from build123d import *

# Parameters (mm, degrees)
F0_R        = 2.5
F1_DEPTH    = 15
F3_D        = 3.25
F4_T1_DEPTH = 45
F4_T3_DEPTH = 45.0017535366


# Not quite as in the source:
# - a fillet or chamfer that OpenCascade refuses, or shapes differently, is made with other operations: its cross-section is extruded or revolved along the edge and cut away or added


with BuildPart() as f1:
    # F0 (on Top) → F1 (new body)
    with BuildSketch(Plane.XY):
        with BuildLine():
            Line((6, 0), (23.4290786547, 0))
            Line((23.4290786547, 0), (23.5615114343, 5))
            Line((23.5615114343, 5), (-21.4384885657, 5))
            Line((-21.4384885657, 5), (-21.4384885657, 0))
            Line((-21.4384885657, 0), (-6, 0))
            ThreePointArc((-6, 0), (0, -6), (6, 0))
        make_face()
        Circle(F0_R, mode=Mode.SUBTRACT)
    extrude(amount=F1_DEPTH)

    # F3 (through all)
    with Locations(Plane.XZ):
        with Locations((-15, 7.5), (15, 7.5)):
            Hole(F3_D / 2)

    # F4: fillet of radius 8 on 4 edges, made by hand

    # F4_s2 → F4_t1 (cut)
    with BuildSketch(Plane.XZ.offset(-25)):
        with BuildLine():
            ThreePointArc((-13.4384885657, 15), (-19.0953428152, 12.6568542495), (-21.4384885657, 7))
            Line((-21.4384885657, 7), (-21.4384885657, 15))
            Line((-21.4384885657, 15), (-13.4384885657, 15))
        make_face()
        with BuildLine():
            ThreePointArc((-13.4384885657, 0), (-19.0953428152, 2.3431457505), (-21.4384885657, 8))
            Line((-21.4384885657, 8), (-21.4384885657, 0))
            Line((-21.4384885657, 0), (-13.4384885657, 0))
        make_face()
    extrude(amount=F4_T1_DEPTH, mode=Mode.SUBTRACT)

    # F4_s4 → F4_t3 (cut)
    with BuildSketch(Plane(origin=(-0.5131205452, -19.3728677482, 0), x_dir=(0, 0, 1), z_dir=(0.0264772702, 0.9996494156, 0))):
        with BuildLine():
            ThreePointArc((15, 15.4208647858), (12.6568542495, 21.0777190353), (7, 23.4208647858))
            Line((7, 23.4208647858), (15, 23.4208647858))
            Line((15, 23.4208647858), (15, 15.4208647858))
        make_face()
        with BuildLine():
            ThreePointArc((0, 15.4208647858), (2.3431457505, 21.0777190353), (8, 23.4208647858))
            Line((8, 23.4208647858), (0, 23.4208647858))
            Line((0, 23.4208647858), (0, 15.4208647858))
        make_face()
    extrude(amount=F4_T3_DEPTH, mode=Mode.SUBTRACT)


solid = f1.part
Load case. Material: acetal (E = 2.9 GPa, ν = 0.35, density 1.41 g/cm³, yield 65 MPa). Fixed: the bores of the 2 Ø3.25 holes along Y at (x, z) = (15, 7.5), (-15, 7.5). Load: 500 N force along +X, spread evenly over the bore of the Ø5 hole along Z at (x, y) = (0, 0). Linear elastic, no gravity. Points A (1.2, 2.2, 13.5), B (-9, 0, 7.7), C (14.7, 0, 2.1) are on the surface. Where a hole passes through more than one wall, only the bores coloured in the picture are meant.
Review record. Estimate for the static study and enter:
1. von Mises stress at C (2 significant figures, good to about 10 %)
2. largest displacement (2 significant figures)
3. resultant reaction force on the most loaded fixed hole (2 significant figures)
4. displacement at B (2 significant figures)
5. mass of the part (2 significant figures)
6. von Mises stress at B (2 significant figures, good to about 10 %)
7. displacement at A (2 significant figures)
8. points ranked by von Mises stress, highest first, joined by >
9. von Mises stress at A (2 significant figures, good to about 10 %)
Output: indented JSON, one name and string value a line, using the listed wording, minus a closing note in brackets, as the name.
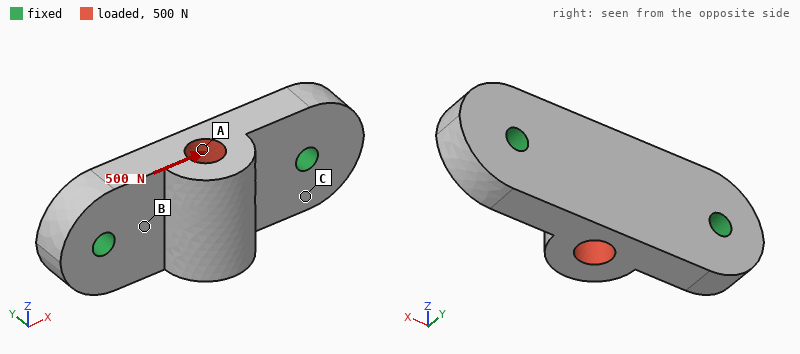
{
  "von Mises stress at C": "1.3 MPa",
  "largest displacement": "35 µm",
  "resultant reaction force on the most loaded fixed hole": "260 N",
  "displacement at B": "10 µm",
  "mass of the part": "5.0 g",
  "von Mises stress at B": "7.3 MPa",
  "displacement at A": "18 µm",
  "points ranked by von Mises stress, highest first, joined by >": "B > A > C",
  "von Mises stress at A": "3.3 MPa"
}
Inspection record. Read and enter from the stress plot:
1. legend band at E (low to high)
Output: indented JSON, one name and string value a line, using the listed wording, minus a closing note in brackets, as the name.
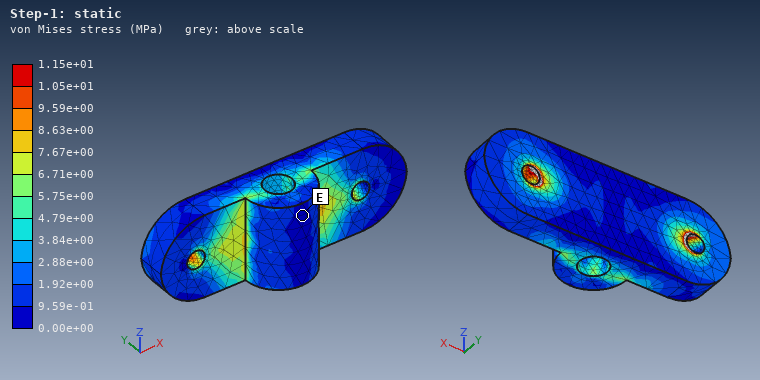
{
  "legend band at E": "0.00e+00 to 9.59e-01 MPa"
}
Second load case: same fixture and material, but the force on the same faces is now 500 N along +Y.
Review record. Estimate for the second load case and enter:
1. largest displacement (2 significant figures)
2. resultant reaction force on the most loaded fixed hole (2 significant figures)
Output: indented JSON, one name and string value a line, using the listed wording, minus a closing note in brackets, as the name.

{
  "largest displacement": "0.15 mm",
  "resultant reaction force on the most loaded fixed hole": "250 N"
}
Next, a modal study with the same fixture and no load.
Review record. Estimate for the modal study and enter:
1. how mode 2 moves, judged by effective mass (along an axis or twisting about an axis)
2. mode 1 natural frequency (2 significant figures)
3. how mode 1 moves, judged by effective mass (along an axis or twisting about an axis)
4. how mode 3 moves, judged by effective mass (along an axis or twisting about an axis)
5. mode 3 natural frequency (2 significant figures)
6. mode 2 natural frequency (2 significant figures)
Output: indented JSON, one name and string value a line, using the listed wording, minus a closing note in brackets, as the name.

{
  "how mode 2 moves, judged by effective mass": "along Y",
  "mode 1 natural frequency": "5600 Hz",
  "how mode 1 moves, judged by effective mass": "along Z",
  "how mode 3 moves, judged by effective mass": "along Z",
  "mode 3 natural frequency": "8600 Hz",
  "mode 2 natural frequency": "6300 Hz"
}
